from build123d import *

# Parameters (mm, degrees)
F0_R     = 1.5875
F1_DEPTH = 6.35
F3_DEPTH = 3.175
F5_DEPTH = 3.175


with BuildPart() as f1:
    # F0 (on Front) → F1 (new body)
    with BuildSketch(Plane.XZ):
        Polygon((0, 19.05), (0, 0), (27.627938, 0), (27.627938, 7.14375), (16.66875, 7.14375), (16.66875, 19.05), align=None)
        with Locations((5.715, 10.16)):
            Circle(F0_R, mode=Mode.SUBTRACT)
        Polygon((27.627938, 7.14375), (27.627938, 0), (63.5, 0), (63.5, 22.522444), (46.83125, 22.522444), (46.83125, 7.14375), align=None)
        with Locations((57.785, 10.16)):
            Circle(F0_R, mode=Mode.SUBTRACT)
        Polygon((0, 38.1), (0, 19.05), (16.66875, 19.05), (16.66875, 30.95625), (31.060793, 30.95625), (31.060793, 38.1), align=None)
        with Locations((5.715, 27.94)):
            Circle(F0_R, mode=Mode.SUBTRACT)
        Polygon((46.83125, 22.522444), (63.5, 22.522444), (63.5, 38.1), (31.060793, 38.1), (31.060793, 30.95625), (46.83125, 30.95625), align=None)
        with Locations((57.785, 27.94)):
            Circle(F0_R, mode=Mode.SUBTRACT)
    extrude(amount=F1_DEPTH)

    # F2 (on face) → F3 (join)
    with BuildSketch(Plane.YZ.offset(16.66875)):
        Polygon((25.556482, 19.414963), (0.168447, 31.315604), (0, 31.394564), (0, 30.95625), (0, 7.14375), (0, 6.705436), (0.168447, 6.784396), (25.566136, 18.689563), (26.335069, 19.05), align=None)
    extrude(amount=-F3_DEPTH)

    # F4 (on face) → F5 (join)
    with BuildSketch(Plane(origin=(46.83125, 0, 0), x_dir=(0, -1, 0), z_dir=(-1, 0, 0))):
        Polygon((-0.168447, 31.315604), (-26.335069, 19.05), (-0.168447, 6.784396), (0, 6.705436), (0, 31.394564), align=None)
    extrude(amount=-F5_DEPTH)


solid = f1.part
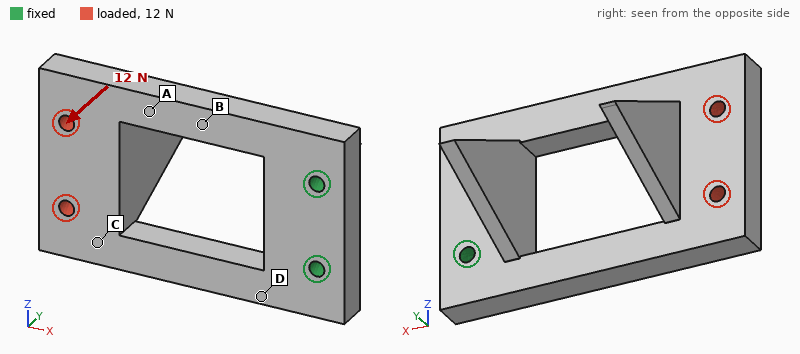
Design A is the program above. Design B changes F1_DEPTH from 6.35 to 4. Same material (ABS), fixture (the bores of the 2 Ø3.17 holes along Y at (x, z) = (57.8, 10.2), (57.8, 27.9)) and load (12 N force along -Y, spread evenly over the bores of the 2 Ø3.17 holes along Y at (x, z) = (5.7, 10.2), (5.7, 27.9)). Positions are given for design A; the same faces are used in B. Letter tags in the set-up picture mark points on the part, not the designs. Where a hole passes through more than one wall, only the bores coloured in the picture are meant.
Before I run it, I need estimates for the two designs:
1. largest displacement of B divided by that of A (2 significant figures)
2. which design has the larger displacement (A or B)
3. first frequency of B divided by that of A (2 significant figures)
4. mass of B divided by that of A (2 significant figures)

3.7
B
0.63
0.69
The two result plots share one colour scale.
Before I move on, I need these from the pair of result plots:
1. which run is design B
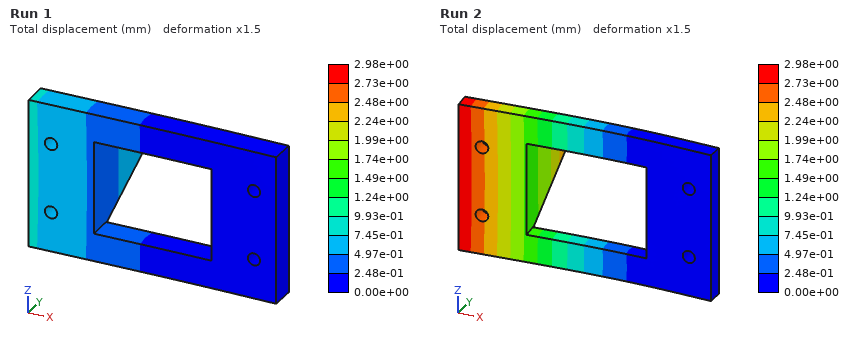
Run 2
